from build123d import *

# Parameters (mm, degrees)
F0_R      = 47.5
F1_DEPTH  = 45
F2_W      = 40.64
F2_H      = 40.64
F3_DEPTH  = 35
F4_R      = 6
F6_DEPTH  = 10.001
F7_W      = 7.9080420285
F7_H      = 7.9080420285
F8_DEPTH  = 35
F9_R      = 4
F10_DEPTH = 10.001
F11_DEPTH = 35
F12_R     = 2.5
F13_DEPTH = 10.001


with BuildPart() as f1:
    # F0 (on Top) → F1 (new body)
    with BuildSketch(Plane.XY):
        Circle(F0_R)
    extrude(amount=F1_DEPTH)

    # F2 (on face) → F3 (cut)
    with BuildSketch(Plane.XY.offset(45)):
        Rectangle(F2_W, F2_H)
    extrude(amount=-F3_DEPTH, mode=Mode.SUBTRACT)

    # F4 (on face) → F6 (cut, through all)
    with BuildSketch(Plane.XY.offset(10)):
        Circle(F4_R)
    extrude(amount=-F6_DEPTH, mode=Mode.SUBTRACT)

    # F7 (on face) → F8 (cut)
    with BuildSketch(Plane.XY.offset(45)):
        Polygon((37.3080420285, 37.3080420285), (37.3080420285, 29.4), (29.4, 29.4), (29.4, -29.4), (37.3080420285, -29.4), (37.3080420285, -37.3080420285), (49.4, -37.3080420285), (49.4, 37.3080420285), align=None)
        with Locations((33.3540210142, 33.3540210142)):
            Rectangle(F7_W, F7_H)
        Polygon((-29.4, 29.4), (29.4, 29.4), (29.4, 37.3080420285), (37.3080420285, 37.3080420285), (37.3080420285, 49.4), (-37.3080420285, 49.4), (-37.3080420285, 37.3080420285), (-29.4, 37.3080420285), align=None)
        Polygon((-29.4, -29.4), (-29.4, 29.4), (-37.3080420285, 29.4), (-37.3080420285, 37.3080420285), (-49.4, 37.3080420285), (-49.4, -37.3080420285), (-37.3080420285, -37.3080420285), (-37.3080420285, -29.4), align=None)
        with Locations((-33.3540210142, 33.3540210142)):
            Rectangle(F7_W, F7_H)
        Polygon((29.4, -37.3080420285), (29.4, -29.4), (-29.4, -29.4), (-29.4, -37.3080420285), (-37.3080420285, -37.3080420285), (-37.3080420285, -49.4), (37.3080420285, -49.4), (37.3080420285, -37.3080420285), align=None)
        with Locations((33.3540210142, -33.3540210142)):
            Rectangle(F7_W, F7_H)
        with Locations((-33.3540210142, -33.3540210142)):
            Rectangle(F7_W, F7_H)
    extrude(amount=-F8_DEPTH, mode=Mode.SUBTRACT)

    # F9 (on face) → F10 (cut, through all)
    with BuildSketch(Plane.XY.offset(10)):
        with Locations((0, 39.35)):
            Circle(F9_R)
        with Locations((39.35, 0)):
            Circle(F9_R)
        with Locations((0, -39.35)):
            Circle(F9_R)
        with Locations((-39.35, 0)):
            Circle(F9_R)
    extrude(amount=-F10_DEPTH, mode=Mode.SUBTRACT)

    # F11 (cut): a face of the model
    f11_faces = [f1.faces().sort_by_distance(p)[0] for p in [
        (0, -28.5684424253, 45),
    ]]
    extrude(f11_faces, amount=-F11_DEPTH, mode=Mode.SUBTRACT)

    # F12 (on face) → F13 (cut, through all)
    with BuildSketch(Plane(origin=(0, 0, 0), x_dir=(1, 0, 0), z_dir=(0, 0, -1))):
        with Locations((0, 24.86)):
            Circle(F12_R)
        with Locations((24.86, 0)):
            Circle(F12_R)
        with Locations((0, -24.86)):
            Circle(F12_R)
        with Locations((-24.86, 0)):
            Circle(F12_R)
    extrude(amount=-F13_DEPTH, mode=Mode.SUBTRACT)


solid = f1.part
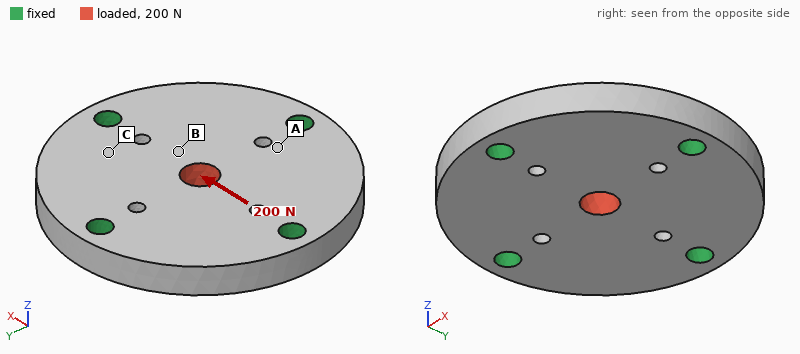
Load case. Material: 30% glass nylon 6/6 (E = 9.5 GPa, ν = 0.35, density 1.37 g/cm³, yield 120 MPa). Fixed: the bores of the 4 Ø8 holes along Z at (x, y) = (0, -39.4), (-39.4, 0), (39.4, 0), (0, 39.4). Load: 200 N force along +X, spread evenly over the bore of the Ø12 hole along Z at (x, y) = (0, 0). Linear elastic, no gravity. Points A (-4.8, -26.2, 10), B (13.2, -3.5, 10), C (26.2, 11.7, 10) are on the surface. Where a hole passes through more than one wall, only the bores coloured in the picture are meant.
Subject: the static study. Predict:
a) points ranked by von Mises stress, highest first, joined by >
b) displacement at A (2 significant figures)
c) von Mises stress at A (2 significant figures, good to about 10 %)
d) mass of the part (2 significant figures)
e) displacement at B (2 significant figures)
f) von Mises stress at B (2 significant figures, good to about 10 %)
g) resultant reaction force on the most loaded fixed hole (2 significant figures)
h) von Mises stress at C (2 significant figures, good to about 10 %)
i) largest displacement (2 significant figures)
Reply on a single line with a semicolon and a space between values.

B > C > A; 0.39 µm; 0.090 MPa; 92 g; 1.0 µm; 0.42 MPa; 65 N; 0.17 MPa; 1.5 µm
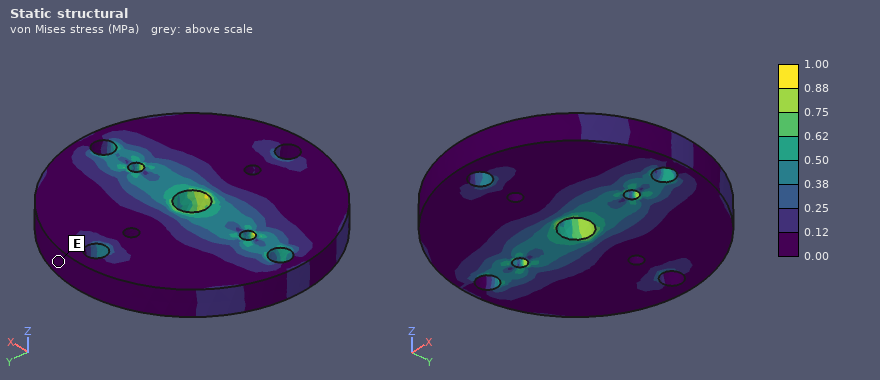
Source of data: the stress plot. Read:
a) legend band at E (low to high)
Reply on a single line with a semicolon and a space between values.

0.00 to 0.12 MPa
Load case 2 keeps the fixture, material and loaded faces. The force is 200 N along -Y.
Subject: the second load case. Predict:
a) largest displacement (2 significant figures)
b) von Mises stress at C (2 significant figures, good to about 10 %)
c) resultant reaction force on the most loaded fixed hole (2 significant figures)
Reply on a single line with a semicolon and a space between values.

1.5 µm; 0.087 MPa; 65 N
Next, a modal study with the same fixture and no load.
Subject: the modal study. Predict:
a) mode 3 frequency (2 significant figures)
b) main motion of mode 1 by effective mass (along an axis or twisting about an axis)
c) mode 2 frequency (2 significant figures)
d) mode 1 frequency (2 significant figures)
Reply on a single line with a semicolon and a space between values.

6700 Hz; along Z; 6400 Hz; 5800 Hz
